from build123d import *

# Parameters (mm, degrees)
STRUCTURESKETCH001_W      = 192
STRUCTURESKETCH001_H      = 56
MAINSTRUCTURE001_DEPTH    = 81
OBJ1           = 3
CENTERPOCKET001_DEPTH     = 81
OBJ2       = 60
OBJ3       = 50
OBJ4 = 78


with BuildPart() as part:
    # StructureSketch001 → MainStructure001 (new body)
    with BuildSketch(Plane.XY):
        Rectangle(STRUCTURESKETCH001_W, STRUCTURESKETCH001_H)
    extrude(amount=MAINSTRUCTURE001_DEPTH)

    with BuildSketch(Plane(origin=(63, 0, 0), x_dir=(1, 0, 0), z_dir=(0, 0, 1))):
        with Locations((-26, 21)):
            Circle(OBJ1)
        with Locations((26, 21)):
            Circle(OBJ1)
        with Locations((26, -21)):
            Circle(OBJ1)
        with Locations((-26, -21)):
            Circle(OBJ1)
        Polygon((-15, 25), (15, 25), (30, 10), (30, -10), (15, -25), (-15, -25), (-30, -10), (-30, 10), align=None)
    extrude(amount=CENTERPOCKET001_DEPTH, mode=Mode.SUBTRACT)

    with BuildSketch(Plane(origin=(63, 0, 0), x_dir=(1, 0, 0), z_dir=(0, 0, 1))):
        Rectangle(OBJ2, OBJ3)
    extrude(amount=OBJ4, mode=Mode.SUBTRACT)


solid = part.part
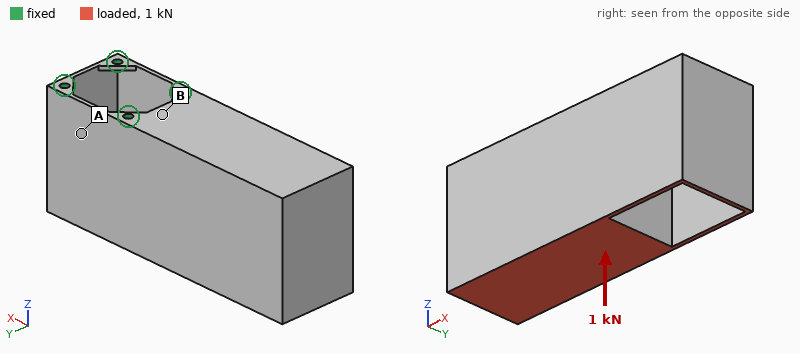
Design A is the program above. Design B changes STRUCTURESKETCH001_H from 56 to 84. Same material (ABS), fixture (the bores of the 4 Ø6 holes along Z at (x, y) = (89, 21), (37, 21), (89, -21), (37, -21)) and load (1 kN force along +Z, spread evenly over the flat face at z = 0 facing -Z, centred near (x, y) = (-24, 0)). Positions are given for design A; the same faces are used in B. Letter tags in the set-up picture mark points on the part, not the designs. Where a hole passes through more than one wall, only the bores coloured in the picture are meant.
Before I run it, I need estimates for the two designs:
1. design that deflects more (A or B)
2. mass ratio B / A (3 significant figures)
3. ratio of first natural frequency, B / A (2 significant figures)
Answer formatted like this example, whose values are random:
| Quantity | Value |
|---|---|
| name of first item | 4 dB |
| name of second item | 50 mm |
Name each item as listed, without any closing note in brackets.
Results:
| Quantity | Value |
|---|---|
| design that deflects more | A |
| mass ratio B / A | 1.69 |
| ratio of first natural frequency, B / A | 1.1 |
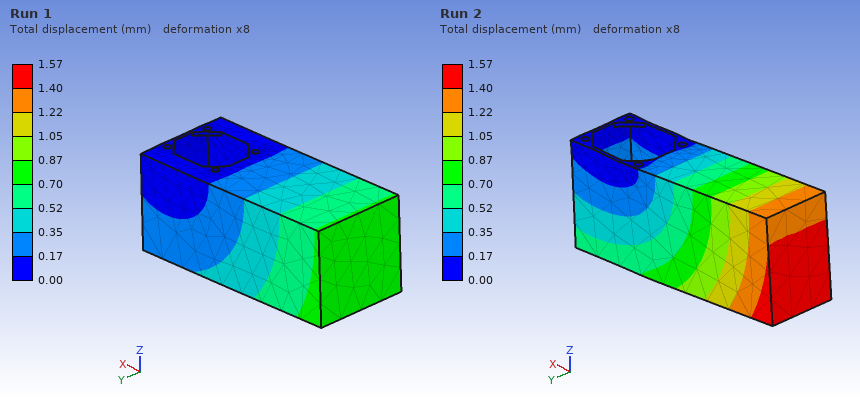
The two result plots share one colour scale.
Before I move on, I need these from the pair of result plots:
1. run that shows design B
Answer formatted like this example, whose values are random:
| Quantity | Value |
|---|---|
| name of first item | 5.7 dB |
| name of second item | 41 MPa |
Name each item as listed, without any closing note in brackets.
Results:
| Quantity | Value |
|---|---|
| run that shows design B | Run 1 |
